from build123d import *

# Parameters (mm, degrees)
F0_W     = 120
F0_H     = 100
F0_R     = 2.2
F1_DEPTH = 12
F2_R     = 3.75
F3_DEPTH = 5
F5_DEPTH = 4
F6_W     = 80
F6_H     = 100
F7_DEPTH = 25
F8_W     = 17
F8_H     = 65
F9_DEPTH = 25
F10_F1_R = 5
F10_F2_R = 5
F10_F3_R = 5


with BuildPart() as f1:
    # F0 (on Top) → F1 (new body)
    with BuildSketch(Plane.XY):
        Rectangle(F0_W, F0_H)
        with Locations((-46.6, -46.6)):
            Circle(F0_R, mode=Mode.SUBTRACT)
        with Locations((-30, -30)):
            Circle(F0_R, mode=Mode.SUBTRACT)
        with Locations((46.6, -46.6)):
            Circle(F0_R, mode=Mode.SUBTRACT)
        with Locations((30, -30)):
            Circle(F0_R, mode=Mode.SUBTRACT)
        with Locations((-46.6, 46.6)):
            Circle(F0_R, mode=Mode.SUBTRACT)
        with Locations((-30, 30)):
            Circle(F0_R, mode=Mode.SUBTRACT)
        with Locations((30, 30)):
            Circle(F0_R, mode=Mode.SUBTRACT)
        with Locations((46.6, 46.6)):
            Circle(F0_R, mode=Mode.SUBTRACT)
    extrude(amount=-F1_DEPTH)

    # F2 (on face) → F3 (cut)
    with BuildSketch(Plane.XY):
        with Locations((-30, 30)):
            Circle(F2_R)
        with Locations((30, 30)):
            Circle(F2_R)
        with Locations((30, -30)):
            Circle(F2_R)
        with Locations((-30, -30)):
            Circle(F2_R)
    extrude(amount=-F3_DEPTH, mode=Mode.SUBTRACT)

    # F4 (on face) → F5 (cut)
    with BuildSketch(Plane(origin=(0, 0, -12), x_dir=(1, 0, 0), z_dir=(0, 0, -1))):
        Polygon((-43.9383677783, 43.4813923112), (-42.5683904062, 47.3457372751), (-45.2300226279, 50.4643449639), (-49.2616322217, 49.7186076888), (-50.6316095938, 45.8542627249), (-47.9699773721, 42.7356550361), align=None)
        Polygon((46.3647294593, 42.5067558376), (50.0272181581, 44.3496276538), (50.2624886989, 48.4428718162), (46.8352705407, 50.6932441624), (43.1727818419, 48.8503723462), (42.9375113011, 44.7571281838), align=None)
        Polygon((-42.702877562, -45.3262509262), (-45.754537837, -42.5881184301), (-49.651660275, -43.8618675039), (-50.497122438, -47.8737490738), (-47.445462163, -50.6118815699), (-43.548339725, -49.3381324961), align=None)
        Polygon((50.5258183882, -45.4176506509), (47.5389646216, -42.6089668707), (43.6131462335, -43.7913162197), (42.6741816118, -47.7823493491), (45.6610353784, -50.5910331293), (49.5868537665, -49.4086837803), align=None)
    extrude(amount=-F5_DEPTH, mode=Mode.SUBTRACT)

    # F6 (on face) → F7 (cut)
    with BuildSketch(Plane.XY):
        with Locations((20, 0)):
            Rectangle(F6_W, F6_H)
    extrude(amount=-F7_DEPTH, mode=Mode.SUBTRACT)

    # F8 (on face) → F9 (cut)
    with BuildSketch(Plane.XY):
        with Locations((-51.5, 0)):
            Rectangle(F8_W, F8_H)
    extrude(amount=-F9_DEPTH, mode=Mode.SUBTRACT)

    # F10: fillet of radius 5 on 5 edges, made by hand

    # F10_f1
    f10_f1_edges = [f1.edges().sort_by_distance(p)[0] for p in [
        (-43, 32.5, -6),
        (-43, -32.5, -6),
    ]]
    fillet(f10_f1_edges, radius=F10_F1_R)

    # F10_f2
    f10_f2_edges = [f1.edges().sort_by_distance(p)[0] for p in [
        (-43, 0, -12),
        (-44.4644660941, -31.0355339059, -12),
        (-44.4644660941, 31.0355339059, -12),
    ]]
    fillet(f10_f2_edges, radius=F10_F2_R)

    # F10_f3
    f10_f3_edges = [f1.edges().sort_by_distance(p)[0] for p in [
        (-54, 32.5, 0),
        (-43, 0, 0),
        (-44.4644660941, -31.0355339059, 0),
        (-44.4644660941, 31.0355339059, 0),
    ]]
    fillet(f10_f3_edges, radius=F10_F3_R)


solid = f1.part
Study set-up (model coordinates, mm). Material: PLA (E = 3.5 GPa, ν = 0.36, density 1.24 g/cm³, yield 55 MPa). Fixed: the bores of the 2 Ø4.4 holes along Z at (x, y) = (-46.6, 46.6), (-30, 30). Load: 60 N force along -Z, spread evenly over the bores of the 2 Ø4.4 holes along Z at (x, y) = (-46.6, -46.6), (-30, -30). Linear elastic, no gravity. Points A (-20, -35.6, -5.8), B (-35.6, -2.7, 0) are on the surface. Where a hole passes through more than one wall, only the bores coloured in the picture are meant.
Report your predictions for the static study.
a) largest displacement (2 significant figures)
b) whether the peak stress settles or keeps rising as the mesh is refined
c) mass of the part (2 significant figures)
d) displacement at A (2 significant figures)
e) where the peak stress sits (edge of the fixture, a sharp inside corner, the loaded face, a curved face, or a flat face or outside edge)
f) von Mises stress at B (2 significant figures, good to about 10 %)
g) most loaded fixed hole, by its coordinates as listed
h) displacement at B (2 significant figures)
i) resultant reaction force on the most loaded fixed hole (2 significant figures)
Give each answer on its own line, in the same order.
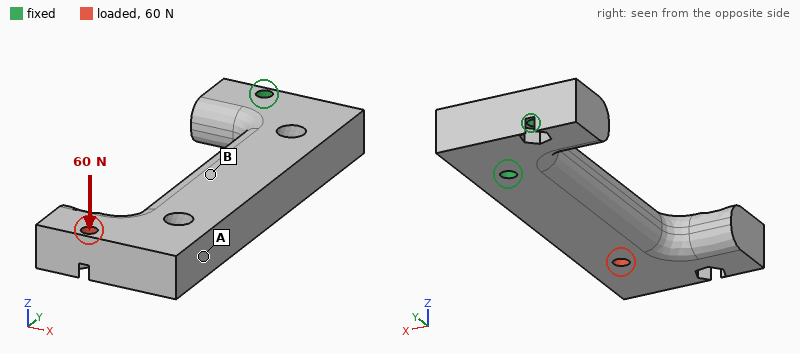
1.2 mm
keeps rising
40 g
0.74 mm
edge of the fixture
4.4 MPa
(-30, 30)
0.31 mm
140 N
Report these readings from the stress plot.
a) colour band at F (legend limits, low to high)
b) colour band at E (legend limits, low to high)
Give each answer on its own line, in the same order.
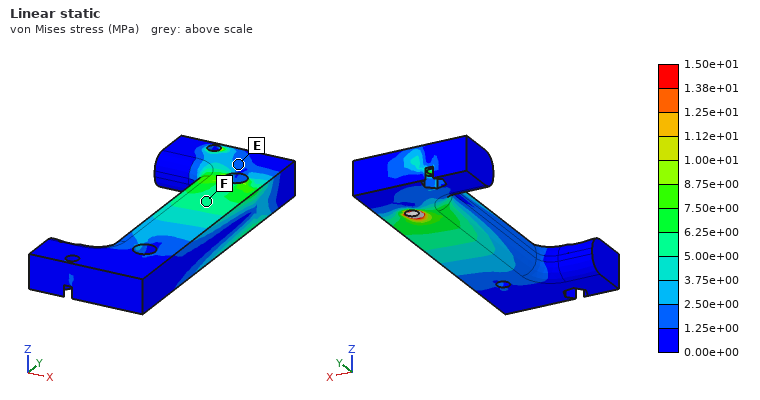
5.00e+00 to 6.25e+00 MPa
1.25e+00 to 2.50e+00 MPa
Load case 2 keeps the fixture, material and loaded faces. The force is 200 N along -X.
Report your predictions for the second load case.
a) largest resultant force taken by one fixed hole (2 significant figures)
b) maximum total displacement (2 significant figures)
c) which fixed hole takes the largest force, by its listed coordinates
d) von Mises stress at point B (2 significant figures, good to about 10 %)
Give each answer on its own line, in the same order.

620 N
1.2 mm
(-30, 30)
3.4 MPa
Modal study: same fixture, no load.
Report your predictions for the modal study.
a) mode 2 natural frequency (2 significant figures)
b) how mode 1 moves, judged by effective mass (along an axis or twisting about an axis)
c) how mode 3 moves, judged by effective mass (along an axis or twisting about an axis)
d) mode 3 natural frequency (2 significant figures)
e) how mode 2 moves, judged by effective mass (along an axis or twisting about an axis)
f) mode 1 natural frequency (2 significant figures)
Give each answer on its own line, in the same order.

610 Hz
along Z
twisting about Y
1400 Hz
along X
350 Hz
